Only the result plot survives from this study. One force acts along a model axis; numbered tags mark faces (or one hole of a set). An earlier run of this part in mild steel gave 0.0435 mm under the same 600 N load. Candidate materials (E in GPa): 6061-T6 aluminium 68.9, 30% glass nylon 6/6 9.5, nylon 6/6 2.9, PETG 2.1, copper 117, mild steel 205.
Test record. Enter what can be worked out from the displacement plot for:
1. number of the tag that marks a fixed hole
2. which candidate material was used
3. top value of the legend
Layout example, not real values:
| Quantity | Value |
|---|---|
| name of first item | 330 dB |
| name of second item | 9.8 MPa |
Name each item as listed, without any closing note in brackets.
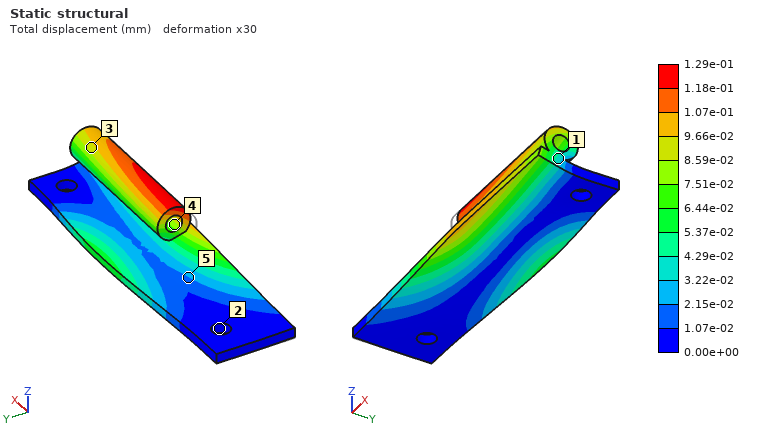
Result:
| Quantity | Value |
|---|---|
| number of the tag that marks a fixed hole | 2 |
| which candidate material was used | 6061-T6 aluminium |
| top value of the legend | 1.29e-01 mm |
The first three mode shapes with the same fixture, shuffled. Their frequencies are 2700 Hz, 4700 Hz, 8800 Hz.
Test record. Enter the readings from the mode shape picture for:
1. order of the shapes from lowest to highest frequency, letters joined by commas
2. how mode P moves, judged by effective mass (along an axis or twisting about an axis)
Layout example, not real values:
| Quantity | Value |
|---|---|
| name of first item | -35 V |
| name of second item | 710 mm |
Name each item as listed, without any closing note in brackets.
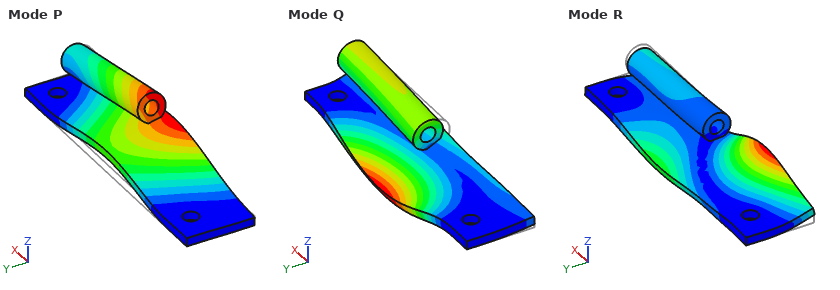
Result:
| Quantity | Value |
|---|---|
| order of the shapes from lowest to highest frequency, letters joined by commas | P, Q, R |
| how mode P moves, judged by effective mass | along Z |
